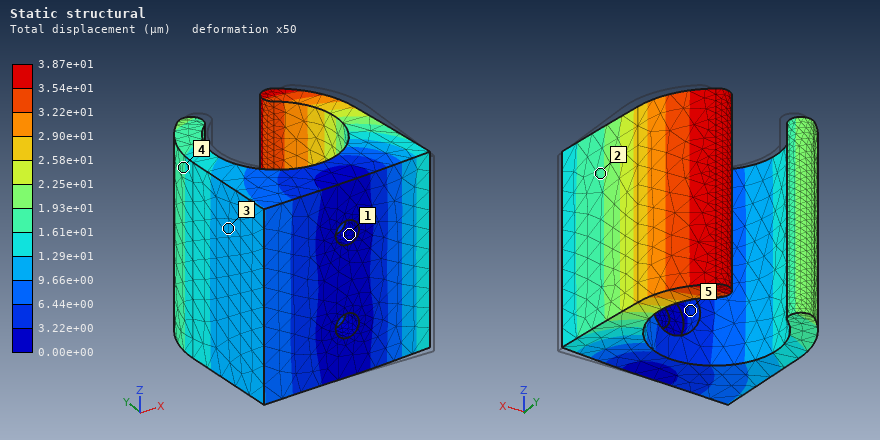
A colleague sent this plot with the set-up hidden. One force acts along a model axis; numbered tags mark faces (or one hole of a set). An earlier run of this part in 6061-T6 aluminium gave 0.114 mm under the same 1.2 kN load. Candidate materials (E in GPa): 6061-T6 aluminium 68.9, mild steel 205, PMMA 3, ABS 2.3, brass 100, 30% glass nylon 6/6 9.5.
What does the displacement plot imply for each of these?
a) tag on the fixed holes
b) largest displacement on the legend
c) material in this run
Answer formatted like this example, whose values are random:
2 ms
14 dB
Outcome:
1
3.87e+01 µm
mild steel
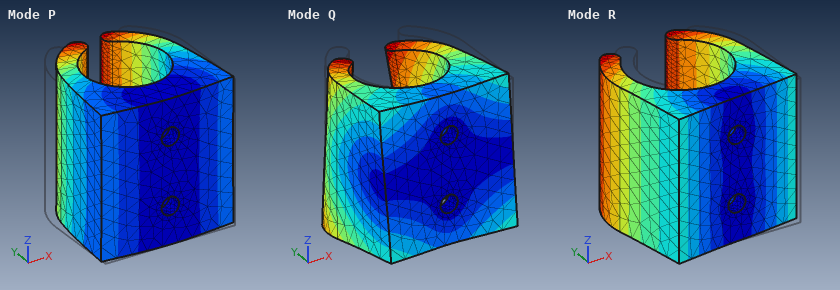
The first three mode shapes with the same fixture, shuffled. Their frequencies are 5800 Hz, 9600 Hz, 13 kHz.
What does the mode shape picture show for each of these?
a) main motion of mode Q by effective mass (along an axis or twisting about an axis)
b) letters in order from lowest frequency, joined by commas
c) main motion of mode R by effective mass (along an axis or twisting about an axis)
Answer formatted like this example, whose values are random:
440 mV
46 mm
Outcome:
along Z
R, P, Q
along X
